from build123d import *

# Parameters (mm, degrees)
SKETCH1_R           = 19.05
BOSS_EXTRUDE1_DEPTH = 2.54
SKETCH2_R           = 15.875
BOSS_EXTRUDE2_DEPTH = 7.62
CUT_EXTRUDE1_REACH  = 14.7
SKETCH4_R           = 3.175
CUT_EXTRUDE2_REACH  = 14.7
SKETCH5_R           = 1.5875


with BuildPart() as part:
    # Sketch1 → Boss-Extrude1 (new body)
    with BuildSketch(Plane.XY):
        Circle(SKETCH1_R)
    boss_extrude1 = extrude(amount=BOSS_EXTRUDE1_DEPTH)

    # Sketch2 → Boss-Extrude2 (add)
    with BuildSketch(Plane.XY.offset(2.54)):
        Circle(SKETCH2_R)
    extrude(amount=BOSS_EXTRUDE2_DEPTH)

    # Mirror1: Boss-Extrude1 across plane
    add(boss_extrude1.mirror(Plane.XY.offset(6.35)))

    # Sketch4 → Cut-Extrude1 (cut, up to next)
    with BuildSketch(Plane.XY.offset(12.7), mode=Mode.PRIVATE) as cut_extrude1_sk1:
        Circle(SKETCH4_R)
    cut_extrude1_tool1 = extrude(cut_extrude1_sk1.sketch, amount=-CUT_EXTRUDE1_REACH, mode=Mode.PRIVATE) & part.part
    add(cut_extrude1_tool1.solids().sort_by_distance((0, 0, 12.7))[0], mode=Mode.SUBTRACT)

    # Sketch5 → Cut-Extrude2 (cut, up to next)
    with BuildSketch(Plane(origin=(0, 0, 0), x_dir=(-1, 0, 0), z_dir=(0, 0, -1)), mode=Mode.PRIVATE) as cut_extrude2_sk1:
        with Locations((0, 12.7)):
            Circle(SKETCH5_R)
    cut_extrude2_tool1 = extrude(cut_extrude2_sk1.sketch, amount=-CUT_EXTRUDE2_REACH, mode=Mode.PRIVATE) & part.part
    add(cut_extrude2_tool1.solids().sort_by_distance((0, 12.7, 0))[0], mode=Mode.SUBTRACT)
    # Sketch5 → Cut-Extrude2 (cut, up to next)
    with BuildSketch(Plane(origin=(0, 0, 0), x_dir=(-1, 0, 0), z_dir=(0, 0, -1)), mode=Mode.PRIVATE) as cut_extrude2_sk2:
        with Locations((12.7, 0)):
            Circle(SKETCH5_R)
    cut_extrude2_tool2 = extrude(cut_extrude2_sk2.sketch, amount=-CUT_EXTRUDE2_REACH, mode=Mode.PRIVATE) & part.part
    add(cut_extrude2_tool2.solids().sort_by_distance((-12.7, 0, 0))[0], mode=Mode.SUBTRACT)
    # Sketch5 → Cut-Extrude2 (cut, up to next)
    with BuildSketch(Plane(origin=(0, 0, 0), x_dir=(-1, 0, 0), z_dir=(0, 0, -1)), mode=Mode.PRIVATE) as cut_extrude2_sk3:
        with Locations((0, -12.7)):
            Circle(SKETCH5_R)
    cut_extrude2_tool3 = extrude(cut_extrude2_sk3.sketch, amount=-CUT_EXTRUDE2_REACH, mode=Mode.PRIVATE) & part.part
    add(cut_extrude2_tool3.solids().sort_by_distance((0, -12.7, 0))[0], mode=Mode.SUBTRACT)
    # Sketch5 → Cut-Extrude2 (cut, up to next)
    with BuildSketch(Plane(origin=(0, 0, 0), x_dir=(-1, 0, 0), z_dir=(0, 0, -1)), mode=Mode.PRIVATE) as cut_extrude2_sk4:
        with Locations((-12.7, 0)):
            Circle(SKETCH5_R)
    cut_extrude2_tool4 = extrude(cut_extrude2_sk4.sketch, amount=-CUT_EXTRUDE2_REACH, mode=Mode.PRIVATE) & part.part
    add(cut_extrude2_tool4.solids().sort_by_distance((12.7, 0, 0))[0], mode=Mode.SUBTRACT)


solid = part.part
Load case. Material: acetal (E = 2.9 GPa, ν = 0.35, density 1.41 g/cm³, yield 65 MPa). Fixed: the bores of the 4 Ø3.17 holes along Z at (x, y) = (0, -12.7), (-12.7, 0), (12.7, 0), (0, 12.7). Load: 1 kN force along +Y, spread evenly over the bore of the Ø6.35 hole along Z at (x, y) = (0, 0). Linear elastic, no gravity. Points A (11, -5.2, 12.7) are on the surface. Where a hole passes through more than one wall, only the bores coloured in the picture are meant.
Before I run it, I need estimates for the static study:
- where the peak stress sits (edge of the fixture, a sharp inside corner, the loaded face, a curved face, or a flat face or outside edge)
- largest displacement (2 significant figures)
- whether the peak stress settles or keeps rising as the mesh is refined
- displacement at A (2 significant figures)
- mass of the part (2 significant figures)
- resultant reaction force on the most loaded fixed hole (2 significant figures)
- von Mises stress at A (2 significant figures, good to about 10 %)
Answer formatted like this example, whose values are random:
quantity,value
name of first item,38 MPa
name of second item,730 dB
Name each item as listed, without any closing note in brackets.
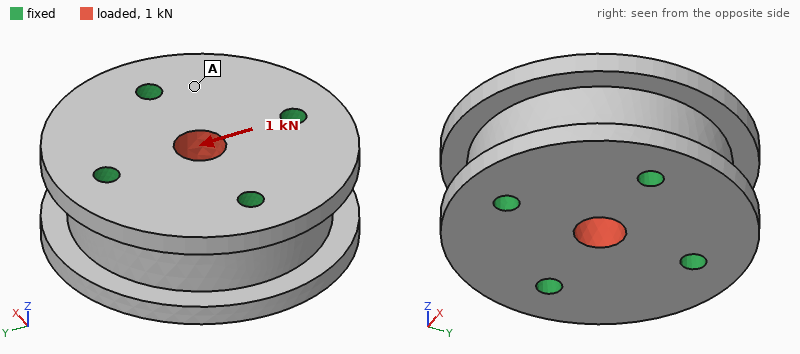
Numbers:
quantity,value
where the peak stress sits,edge of the fixture
largest displacement,13 µm
whether the peak stress settles or keeps rising as the mesh is refined,keeps rising
displacement at A,3.2 µm
mass of the part,16 g
resultant reaction force on the most loaded fixed hole,340 N
von Mises stress at A,1.1 MPa
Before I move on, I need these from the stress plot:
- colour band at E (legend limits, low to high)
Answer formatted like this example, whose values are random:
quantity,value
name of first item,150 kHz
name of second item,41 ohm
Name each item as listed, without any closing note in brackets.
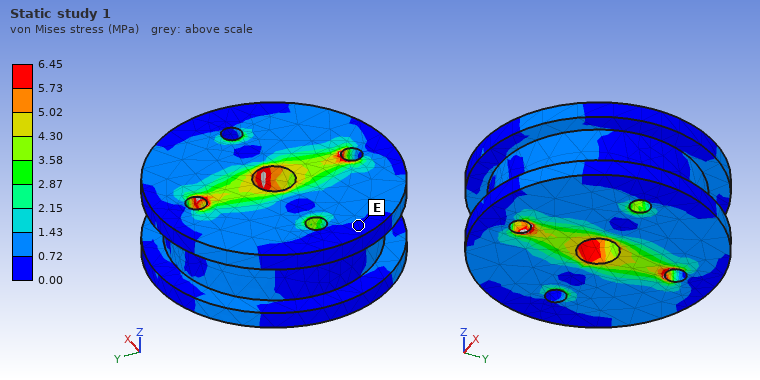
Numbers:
quantity,value
colour band at E,0.00 to 0.72 MPa
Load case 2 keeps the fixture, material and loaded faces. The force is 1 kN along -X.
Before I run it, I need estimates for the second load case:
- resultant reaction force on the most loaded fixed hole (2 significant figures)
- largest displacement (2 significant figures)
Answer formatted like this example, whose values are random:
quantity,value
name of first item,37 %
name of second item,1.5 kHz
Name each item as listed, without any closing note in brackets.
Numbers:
quantity,value
resultant reaction force on the most loaded fixed hole,340 N
largest displacement,13 µm
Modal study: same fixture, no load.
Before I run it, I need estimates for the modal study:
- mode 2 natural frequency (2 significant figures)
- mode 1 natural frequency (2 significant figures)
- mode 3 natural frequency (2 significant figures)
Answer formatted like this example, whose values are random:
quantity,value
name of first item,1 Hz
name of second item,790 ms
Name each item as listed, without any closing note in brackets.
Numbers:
quantity,value
mode 2 natural frequency,15 kHz
mode 1 natural frequency,15 kHz
mode 3 natural frequency,15 kHz
